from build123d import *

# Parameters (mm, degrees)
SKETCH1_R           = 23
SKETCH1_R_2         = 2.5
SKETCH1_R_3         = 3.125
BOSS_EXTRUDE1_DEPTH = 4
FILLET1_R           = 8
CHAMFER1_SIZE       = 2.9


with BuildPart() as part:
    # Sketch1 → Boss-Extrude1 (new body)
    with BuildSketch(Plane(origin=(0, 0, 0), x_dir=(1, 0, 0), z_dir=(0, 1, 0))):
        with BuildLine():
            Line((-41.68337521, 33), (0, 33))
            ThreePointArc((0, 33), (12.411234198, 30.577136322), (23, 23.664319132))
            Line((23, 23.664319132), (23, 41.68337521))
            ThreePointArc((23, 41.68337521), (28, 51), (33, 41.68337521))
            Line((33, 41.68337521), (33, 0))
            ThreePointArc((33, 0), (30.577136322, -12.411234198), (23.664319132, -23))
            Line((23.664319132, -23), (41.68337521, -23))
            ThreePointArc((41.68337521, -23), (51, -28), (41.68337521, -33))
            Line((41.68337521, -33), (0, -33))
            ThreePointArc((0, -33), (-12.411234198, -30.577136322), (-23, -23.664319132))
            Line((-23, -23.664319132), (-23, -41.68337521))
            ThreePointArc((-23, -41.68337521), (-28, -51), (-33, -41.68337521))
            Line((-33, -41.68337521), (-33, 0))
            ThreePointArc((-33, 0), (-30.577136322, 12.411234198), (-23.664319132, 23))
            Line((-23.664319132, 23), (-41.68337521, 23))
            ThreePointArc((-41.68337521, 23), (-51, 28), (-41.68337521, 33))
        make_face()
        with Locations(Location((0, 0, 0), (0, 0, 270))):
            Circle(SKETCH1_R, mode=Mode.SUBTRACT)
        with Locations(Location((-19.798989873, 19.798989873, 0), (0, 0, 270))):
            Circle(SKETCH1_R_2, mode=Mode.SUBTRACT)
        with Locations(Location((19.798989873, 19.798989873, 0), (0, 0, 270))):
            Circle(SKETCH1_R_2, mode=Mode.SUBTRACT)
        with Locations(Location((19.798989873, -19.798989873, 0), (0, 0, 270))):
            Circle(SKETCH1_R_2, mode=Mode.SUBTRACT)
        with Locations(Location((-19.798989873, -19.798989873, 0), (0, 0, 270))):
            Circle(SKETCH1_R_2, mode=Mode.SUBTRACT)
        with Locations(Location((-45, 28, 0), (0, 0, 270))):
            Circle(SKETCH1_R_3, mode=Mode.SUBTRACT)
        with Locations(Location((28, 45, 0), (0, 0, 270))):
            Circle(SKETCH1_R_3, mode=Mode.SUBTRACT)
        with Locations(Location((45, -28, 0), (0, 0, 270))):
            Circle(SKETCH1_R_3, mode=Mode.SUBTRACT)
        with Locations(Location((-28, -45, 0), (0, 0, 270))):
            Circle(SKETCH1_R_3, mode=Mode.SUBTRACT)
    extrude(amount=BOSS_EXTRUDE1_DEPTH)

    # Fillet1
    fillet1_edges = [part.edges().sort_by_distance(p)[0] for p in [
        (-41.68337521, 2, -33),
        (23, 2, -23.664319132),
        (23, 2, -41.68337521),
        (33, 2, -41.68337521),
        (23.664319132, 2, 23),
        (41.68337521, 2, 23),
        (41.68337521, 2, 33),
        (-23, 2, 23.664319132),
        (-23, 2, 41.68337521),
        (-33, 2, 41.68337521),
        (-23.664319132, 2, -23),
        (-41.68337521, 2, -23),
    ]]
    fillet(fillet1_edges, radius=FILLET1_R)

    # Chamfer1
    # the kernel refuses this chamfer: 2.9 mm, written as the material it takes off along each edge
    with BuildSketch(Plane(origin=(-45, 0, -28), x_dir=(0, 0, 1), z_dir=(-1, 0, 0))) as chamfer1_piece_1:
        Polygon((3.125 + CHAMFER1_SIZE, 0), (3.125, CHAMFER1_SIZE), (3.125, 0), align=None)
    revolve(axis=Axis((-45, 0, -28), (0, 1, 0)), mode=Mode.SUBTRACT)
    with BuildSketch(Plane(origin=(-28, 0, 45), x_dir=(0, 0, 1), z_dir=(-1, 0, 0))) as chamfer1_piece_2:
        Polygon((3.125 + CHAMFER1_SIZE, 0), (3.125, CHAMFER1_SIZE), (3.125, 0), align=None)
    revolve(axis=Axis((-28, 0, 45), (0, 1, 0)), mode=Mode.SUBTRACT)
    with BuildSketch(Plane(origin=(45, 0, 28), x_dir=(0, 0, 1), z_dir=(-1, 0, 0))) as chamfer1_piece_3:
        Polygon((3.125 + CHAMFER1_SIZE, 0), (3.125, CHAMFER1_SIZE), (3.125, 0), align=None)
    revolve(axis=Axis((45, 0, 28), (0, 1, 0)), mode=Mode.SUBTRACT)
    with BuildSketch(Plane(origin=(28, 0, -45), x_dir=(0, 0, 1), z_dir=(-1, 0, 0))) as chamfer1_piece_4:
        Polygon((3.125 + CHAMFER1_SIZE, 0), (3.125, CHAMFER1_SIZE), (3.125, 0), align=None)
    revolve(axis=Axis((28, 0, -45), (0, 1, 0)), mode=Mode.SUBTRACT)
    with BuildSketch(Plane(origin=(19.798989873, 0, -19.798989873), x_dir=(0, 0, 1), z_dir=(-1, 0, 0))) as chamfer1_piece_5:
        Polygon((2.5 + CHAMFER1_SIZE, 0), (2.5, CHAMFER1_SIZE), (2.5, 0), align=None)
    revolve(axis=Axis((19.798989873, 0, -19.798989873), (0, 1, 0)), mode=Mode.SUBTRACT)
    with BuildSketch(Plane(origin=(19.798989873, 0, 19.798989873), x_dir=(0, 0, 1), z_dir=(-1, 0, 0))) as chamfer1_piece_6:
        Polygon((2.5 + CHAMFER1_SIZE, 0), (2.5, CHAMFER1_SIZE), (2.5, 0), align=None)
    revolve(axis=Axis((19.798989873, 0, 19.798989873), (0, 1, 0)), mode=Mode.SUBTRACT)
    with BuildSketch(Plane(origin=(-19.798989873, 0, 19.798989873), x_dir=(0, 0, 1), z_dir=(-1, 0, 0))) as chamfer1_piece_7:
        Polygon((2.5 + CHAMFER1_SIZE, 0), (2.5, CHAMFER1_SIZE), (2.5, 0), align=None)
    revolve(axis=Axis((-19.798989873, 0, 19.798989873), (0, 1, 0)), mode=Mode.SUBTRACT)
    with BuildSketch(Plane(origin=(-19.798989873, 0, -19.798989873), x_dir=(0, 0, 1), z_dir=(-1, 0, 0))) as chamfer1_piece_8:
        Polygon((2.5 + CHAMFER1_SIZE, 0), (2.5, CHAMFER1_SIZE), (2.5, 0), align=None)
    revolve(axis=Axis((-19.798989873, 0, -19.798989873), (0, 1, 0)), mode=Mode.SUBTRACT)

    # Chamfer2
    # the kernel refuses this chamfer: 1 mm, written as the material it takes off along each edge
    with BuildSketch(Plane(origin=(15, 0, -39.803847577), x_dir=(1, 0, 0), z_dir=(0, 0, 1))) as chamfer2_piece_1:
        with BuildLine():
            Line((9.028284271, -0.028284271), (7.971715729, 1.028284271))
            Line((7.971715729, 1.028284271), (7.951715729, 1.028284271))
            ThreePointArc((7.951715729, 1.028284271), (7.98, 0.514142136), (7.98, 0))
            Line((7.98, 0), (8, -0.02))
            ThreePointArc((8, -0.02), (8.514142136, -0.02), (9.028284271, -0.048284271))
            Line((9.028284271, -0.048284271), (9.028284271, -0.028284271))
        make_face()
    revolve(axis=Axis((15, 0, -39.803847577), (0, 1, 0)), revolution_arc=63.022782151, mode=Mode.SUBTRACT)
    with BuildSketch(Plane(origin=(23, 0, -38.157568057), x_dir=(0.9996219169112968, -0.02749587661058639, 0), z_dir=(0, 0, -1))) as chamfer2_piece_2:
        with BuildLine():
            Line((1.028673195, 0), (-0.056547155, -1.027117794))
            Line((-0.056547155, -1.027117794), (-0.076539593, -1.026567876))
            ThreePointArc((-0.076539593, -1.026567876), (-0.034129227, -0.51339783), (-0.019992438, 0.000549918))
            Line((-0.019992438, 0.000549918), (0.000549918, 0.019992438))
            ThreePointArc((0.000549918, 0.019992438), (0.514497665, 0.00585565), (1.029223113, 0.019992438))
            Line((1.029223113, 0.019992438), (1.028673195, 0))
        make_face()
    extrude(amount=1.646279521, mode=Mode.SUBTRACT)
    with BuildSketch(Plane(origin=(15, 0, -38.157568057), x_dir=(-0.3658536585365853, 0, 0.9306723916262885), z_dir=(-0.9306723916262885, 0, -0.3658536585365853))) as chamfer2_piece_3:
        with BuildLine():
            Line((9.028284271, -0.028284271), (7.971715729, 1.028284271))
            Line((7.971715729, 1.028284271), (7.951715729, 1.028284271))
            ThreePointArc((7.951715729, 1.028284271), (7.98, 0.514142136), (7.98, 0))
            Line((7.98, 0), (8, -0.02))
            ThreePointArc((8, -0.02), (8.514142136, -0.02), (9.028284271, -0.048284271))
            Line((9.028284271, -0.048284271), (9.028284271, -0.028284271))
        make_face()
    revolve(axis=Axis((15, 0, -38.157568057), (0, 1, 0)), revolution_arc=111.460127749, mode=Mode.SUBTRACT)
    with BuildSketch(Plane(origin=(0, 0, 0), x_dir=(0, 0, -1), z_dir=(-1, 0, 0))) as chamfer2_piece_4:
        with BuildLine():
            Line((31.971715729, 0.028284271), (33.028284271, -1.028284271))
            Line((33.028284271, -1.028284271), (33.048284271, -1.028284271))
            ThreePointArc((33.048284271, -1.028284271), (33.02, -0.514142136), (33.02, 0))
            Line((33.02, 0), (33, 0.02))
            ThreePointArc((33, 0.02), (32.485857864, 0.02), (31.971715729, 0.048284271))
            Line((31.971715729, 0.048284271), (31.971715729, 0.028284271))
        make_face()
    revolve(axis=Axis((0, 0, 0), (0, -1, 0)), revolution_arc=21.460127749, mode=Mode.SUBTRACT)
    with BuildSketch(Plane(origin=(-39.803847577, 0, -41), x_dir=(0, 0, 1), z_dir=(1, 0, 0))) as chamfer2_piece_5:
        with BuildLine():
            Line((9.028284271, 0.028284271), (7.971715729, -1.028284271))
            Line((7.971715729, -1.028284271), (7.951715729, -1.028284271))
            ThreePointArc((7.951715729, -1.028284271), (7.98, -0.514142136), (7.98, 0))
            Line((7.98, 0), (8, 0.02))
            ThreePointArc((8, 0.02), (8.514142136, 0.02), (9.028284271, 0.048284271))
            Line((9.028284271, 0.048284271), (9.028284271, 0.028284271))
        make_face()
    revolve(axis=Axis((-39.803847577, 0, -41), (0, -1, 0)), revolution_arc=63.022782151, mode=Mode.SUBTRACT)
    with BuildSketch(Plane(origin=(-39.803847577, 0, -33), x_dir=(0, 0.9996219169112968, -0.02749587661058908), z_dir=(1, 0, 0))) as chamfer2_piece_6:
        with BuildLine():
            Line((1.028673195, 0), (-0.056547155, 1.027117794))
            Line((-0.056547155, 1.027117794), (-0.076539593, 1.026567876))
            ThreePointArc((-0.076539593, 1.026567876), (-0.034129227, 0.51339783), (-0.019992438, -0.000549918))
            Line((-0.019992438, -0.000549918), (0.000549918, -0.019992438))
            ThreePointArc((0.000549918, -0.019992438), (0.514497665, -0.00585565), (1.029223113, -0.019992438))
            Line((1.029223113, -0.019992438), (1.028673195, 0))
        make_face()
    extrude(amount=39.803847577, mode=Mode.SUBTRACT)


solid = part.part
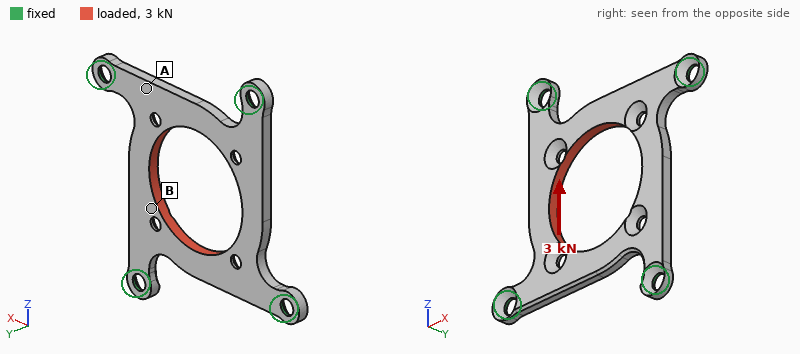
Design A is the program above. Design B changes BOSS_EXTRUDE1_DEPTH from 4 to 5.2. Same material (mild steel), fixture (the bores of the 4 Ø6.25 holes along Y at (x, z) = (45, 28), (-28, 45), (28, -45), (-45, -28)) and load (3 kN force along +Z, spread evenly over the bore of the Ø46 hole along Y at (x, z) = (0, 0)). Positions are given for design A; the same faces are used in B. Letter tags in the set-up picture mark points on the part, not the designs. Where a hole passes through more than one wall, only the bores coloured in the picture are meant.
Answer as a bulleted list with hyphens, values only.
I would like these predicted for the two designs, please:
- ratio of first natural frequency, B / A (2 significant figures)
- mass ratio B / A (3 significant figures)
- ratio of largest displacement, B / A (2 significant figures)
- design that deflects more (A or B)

- 1.3
- 1.32
- 0.64
- A
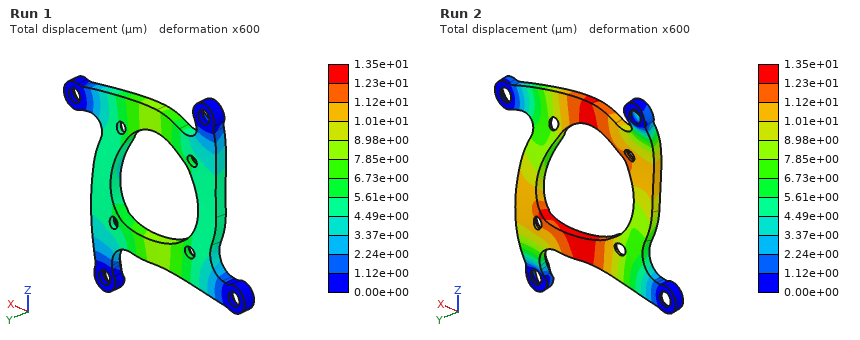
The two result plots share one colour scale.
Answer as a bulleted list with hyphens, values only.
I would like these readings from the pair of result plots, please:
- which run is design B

- Run 1
